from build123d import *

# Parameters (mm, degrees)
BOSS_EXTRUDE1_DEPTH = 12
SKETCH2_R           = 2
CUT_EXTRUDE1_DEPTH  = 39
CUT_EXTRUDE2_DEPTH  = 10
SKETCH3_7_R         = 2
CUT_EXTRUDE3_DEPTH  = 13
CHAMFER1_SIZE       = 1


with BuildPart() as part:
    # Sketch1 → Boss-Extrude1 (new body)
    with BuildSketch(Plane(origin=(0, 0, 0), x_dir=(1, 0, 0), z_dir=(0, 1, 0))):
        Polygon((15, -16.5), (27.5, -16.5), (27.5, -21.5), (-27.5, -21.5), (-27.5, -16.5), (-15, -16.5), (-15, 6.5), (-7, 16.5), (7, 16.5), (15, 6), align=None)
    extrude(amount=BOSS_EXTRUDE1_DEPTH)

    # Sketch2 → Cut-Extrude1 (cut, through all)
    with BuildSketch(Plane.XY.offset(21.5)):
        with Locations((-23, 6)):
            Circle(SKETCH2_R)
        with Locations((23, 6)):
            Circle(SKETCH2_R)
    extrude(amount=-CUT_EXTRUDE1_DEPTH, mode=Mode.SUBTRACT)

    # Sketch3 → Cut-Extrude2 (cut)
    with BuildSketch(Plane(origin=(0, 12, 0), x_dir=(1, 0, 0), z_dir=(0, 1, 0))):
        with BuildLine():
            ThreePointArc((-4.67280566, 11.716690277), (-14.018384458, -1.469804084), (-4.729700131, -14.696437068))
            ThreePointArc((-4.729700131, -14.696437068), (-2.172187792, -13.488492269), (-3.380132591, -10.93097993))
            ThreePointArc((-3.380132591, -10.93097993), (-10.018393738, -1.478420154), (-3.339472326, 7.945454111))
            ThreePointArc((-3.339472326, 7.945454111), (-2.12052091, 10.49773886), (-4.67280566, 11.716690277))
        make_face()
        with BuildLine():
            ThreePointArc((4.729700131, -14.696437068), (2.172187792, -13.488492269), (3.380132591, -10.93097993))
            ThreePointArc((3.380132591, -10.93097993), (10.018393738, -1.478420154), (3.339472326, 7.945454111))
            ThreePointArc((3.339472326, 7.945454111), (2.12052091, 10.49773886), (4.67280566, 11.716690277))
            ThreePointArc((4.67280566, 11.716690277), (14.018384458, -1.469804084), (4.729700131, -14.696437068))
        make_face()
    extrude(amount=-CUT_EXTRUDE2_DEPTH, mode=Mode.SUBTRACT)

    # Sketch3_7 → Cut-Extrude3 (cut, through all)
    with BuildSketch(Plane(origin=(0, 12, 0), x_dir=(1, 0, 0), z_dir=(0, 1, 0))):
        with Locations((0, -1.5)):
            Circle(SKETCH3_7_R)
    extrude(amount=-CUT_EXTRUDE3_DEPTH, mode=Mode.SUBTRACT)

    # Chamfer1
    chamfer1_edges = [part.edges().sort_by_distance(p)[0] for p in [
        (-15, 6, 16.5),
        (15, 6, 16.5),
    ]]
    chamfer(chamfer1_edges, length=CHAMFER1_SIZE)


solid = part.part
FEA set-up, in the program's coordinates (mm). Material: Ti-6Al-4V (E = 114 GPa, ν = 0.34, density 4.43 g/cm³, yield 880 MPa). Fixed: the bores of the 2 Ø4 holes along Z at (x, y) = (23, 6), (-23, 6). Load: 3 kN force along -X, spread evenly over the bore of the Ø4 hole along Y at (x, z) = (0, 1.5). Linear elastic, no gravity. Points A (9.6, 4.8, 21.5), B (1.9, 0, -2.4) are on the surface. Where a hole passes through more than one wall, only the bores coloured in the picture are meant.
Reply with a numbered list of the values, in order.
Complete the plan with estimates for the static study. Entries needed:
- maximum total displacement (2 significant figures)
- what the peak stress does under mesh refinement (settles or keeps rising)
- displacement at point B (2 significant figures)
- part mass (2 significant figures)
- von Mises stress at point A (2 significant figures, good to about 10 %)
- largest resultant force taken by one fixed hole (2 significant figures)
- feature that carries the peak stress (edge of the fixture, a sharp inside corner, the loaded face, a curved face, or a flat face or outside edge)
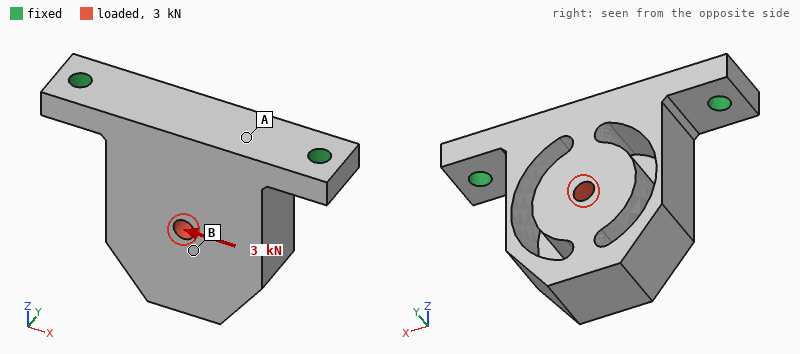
1. 63 µm
2. keeps rising
3. 30 µm
4. 50 g
5. 34 MPa
6. 2.1 kN
7. edge of the fixture
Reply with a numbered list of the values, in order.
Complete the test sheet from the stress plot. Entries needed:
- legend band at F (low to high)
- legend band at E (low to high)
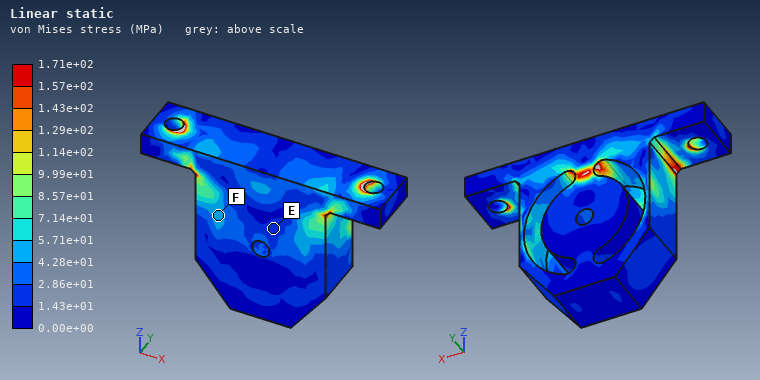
1. 4.28e+01 to 5.71e+01 MPa
2. 1.43e+01 to 2.86e+01 MPa
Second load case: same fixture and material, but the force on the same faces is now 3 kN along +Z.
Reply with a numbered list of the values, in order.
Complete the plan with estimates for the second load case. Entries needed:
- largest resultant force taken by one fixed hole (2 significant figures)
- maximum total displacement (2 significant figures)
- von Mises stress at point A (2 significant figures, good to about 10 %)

1. 1.7 kN
2. 34 µm
3. 35 MPa
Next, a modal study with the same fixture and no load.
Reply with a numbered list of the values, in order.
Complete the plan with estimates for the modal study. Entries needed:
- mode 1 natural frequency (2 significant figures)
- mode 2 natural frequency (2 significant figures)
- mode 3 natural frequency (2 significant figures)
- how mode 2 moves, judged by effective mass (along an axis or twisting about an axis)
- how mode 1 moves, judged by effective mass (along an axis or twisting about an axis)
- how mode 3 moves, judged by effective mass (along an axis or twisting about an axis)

1. 2500 Hz
2. 6800 Hz
3. 8900 Hz
4. along X
5. along Y
6. along Z
